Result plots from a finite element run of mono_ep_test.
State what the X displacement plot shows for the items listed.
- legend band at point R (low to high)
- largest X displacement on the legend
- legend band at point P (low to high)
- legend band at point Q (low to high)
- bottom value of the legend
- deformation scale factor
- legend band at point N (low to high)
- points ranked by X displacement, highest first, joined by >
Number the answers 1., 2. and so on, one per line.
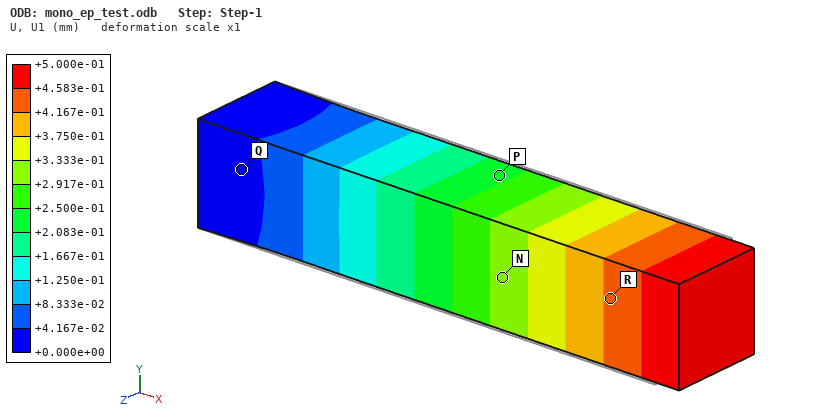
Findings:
1. +4.167e-01 to +4.583e-01 mm
2. +5.000e-01 mm
3. +2.083e-01 to +2.500e-01 mm
4. +0.000e+00 to +4.167e-02 mm
5. +0.000e+00 mm
6. 1
7. +2.917e-01 to +3.333e-01 mm
8. R > N > P > Q
